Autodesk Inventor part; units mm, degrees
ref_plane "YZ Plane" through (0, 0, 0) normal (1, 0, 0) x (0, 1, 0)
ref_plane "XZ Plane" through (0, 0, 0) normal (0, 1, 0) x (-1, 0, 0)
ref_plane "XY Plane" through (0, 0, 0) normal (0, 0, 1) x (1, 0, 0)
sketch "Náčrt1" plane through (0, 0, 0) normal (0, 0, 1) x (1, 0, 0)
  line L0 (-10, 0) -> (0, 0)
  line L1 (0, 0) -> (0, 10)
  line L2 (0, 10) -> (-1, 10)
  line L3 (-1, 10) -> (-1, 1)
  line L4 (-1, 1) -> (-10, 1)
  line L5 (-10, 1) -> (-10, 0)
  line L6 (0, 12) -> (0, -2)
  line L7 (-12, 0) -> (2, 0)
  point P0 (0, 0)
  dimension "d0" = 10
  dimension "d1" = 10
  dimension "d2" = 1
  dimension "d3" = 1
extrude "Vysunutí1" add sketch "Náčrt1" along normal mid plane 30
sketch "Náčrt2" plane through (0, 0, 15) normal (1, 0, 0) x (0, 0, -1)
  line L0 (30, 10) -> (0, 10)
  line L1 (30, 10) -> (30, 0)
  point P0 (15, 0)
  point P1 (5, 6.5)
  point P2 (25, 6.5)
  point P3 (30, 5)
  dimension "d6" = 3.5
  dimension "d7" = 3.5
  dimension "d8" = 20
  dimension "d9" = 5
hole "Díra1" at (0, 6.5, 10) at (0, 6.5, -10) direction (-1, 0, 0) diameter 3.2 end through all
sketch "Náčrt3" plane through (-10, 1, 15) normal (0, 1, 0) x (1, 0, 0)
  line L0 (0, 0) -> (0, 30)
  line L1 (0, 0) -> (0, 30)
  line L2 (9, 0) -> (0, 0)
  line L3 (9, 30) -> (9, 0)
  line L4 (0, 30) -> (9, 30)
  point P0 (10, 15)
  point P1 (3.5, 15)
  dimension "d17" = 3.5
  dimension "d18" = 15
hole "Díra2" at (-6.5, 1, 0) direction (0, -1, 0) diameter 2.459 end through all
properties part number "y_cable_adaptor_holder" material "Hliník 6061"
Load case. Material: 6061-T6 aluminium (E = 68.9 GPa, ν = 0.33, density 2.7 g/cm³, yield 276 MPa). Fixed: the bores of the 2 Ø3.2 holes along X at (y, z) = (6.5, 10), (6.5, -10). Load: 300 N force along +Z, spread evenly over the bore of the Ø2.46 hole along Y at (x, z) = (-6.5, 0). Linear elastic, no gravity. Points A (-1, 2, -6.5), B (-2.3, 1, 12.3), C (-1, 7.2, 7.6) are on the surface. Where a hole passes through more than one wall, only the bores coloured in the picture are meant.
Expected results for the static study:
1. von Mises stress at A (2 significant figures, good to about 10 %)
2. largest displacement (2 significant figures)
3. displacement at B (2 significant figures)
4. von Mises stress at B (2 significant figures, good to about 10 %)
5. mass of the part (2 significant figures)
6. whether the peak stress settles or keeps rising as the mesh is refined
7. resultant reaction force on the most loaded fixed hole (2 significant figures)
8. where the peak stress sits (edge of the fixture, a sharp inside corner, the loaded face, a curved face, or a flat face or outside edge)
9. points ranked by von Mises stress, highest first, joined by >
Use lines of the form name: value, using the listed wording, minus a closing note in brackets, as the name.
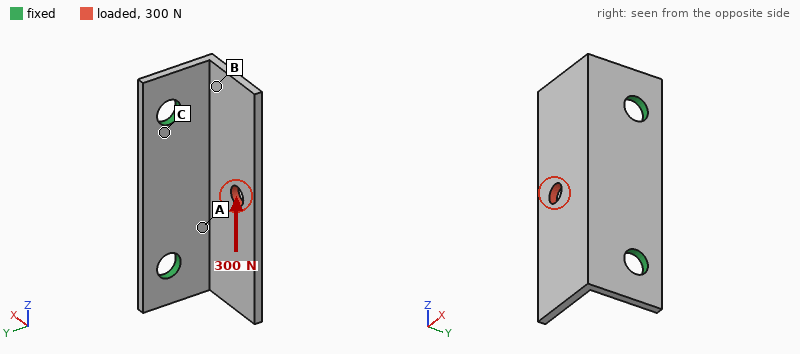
von Mises stress at A: 82 MPa
largest displacement: 0.12 mm
displacement at B: 0.051 mm
von Mises stress at B: 53 MPa
mass of the part: 1.5 g
whether the peak stress settles or keeps rising as the mesh is refined: keeps rising
resultant reaction force on the most loaded fixed hole: 190 N
where the peak stress sits: edge of the fixture
points ranked by von Mises stress, highest first, joined by >: A > B > C
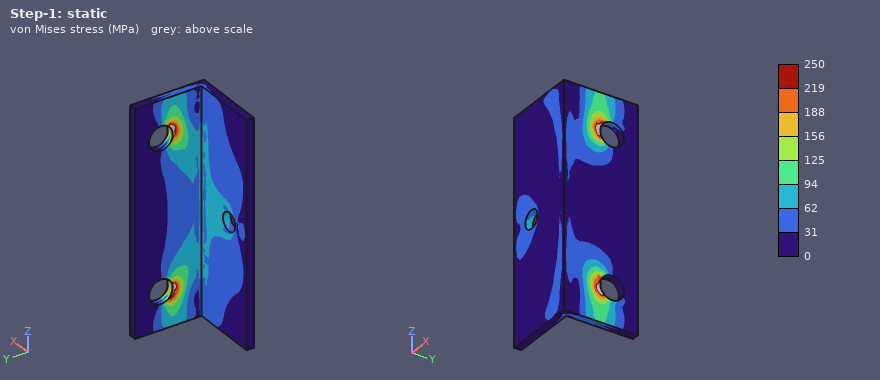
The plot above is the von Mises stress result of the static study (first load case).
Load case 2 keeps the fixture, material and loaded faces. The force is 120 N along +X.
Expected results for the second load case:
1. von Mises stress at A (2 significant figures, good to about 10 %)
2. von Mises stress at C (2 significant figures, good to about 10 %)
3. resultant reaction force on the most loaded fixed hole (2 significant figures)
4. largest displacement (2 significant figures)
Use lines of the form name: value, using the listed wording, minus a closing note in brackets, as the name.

von Mises stress at A: 41 MPa
von Mises stress at C: 41 MPa
resultant reaction force on the most loaded fixed hole: 62 N
largest displacement: 0.11 mm
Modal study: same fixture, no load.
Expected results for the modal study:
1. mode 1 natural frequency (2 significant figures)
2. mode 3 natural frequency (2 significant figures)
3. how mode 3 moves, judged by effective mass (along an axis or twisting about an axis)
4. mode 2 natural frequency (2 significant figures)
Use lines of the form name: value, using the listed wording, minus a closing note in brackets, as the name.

mode 1 natural frequency: 4800 Hz
mode 3 natural frequency: 13 kHz
how mode 3 moves, judged by effective mass: along X
mode 2 natural frequency: 7200 Hz
